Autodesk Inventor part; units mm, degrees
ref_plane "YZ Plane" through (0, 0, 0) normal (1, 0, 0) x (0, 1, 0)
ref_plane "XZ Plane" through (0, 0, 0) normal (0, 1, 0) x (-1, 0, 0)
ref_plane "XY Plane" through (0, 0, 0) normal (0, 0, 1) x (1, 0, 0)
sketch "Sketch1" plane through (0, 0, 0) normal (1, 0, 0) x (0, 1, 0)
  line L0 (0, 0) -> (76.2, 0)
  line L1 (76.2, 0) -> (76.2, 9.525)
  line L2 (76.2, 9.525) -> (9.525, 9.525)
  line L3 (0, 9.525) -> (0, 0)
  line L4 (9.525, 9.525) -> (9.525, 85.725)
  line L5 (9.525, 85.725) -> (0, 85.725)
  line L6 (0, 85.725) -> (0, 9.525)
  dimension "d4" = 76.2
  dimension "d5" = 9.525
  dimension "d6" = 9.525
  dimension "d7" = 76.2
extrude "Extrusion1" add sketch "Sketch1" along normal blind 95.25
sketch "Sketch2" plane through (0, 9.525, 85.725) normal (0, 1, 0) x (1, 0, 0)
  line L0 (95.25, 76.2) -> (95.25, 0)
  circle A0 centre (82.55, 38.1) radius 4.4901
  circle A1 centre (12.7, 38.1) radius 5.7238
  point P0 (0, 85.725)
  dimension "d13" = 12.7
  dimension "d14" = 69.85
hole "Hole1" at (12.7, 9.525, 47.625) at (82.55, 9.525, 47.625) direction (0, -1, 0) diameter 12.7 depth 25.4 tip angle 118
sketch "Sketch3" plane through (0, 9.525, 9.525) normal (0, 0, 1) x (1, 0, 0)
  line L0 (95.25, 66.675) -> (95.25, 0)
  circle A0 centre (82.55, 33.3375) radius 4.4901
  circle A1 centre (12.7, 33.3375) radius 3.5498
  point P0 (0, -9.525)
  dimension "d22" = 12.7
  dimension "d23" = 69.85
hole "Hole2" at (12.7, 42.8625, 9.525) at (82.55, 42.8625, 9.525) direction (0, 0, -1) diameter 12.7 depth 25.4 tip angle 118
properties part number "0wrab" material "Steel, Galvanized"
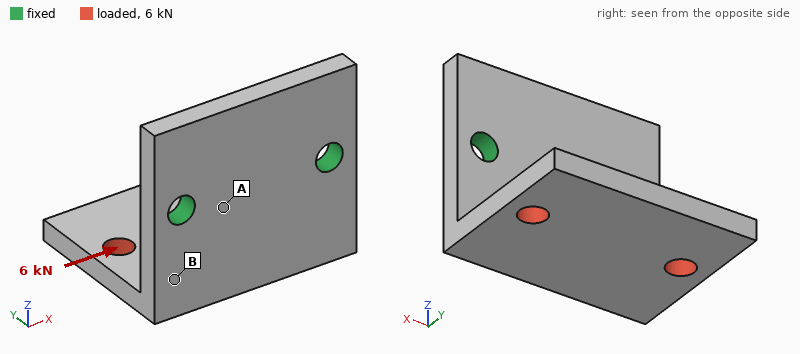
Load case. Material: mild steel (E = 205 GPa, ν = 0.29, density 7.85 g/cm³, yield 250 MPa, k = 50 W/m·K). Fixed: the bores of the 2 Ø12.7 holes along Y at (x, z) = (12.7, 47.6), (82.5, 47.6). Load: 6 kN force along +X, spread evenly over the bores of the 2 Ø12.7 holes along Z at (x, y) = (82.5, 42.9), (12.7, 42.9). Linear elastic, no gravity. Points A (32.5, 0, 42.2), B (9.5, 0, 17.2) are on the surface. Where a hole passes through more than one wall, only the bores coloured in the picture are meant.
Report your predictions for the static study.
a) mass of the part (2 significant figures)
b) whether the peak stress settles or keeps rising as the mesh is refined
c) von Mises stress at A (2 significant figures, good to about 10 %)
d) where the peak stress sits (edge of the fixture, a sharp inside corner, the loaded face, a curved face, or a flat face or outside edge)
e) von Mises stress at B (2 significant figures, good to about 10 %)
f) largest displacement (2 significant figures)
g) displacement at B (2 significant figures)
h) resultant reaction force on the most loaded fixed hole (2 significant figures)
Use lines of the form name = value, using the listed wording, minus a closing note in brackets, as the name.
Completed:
mass of the part = 1.0 kg
whether the peak stress settles or keeps rising as the mesh is refined = keeps rising
von Mises stress at A = 23 MPa
where the peak stress sits = edge of the fixture
von Mises stress at B = 49 MPa
largest displacement = 0.14 mm
displacement at B = 0.036 mm
resultant reaction force on the most loaded fixed hole = 5.4 kN
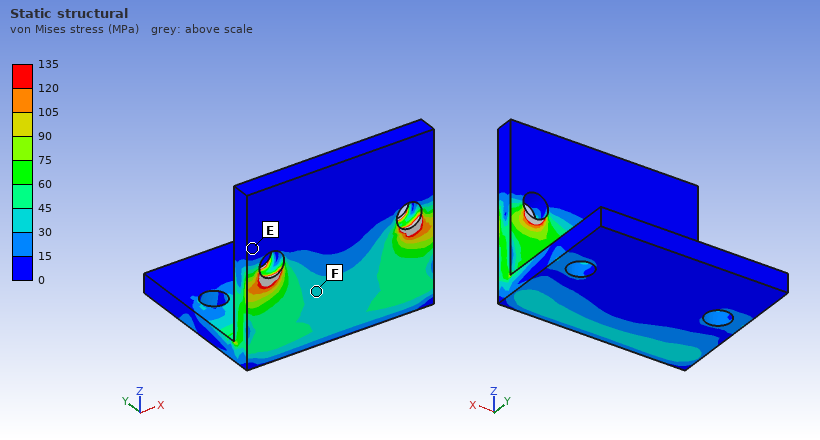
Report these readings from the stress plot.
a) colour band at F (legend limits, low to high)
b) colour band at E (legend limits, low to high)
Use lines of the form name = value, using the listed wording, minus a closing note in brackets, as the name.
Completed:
colour band at F = 30 to 45 MPa
colour band at E = 0 to 15 MPa
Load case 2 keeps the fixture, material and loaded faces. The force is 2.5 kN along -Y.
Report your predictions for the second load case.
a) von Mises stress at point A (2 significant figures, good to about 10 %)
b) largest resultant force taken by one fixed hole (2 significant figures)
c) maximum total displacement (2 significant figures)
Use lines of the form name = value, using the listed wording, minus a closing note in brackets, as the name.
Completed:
von Mises stress at point A = 33 MPa
largest resultant force taken by one fixed hole = 1.3 kN
maximum total displacement = 0.12 mm
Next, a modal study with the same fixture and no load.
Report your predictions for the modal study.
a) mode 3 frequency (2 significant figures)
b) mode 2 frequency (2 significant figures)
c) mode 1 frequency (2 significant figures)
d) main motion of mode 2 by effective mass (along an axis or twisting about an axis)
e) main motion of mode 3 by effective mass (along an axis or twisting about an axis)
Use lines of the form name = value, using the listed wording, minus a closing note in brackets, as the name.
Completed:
mode 3 frequency = 2400 Hz
mode 2 frequency = 1700 Hz
mode 1 frequency = 810 Hz
main motion of mode 2 by effective mass = along X
main motion of mode 3 by effective mass = along Y
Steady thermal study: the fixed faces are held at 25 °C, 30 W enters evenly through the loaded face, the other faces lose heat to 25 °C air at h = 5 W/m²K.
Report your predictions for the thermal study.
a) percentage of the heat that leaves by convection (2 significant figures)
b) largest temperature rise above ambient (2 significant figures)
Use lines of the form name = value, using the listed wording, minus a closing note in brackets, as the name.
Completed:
percentage of the heat that leaves by convection = 13 %
largest temperature rise above ambient = 55 K
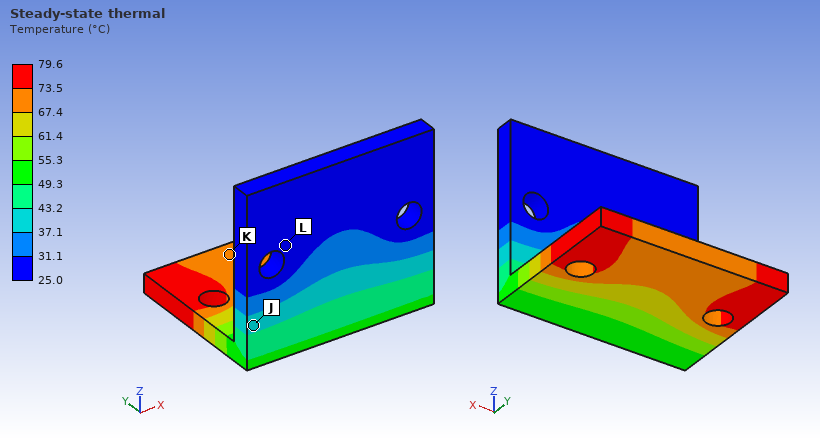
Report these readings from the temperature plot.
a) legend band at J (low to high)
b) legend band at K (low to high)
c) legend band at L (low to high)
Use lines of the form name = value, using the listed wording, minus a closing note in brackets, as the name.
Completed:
legend band at J = 37.1 to 43.2 °C
legend band at K = 67.4 to 73.5 °C
legend band at L = 25.0 to 31.1 °C
